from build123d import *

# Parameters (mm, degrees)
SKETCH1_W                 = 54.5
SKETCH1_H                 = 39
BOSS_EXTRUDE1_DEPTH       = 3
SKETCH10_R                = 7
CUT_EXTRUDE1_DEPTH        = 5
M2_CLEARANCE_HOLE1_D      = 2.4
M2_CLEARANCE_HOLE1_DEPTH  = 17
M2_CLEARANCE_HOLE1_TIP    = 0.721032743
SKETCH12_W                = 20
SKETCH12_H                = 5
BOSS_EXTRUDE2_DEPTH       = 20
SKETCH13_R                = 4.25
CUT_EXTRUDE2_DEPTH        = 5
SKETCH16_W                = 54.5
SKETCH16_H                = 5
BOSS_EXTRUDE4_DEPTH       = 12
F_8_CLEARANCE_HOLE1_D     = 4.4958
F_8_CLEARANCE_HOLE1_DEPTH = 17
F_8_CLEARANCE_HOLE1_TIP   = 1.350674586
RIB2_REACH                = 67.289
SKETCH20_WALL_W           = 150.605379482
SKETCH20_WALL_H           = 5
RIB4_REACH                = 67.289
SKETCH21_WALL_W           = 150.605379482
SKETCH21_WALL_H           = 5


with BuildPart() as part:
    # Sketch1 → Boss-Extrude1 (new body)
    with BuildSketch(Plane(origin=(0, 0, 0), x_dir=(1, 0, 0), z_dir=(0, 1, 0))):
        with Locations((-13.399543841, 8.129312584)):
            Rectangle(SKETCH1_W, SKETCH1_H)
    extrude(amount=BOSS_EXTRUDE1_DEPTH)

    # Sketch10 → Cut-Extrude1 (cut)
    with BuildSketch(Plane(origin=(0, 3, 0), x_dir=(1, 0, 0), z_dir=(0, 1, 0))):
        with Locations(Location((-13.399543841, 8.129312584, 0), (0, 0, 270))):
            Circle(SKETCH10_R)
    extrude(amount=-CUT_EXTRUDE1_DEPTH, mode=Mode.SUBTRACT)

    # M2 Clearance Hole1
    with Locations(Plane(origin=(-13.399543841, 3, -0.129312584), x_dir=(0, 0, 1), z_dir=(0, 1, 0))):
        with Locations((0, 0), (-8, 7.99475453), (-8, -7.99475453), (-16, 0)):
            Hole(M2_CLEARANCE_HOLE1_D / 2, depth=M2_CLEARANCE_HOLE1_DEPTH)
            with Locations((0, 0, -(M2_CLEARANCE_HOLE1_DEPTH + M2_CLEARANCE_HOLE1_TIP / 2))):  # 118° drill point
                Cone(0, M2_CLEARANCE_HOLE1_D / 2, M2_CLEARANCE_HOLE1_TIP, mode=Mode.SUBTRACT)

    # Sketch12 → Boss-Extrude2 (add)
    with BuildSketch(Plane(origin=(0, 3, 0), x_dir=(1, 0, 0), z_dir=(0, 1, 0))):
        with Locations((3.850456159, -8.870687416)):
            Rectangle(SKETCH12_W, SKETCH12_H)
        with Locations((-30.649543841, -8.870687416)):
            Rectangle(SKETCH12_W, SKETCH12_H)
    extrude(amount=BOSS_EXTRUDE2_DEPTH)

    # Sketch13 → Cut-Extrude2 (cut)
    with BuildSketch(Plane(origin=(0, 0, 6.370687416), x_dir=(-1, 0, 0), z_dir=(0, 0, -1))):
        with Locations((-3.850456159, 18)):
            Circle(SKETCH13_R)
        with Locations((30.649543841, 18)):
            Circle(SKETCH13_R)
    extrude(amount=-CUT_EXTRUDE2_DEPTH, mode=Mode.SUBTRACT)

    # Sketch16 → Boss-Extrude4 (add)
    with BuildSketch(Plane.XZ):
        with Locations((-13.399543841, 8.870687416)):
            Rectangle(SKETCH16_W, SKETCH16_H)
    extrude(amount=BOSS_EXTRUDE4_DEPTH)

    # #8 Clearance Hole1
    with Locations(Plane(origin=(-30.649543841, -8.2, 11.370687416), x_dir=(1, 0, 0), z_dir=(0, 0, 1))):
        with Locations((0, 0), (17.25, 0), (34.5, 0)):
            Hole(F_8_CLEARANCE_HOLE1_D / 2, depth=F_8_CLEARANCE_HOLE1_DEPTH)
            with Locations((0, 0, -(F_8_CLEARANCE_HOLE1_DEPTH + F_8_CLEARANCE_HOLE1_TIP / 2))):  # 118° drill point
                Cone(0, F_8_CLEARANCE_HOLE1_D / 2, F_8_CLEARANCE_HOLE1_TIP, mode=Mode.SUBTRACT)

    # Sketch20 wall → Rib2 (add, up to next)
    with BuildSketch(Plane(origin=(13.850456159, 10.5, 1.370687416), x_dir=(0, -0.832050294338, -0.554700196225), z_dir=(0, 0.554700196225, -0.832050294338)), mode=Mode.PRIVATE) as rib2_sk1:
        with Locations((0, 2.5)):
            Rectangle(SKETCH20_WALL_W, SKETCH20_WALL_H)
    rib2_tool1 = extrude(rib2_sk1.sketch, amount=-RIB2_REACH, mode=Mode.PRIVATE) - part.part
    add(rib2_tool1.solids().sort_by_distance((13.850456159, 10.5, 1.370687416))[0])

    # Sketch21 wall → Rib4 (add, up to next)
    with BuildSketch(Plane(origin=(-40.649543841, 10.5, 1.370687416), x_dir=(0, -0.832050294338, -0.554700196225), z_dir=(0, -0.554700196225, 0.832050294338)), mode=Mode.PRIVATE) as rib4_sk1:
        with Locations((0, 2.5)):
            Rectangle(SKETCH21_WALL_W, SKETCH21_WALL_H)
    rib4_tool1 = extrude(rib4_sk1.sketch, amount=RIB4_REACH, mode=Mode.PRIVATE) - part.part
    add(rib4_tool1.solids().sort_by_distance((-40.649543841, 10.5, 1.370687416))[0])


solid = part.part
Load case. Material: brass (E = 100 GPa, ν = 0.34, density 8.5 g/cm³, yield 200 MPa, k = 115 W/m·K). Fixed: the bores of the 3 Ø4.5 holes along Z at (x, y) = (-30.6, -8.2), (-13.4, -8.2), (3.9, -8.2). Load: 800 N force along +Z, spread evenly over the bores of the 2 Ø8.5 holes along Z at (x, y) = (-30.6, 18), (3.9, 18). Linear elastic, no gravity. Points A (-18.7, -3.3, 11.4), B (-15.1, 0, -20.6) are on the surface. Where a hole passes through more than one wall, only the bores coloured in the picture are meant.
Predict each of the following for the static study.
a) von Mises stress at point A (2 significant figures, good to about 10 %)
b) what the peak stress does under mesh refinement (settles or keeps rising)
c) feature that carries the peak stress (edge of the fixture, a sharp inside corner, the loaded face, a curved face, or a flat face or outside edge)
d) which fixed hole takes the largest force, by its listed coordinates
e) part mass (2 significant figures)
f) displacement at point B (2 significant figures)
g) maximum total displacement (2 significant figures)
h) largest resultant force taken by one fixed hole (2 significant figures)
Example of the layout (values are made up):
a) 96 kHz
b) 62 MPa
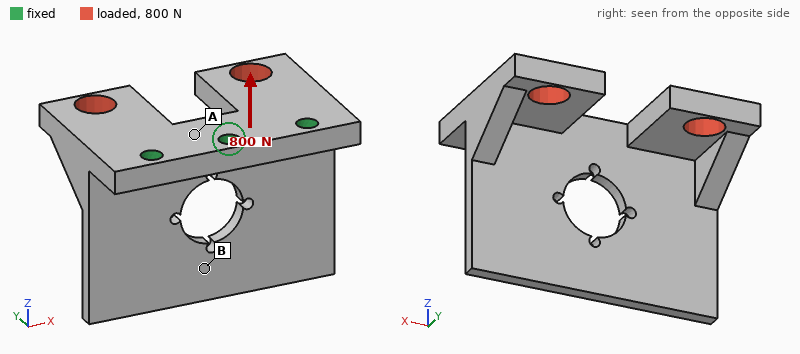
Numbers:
a) 47 MPa
b) keeps rising
c) edge of the fixture
d) (-13.4, -8.2)
e) 110 g
f) 0.094 mm
g) 0.13 mm
h) 370 N
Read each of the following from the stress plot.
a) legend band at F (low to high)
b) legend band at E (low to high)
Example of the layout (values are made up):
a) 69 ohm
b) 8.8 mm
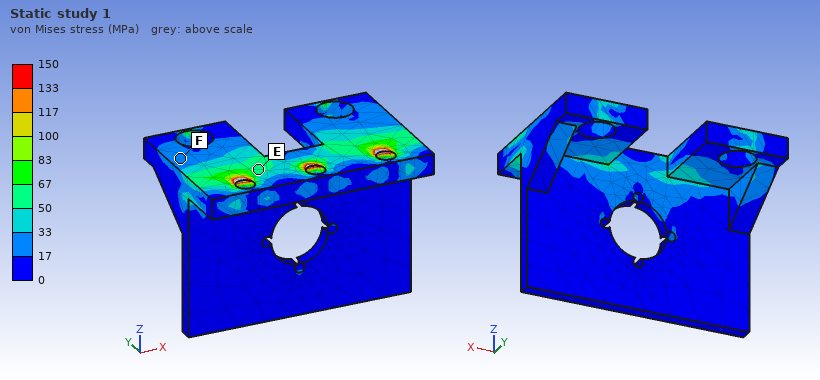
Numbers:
a) 17 to 33 MPa
b) 50 to 67 MPa
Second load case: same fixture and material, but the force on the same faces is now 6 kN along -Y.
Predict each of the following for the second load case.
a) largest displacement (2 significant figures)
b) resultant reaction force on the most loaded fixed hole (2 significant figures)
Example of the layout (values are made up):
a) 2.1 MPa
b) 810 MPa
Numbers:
a) 29 µm
b) 2.6 kN
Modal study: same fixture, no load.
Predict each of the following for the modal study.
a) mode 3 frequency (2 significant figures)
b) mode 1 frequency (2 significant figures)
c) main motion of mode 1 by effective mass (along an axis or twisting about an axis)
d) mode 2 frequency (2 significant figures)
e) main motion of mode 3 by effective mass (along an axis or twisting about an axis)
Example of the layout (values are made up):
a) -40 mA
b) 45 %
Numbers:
a) 3800 Hz
b) 1400 Hz
c) along Y
d) 2400 Hz
e) along Z
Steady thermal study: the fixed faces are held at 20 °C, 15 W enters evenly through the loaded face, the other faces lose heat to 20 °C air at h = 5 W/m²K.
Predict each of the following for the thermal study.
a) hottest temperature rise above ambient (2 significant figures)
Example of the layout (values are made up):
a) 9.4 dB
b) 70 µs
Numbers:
a) 20 K
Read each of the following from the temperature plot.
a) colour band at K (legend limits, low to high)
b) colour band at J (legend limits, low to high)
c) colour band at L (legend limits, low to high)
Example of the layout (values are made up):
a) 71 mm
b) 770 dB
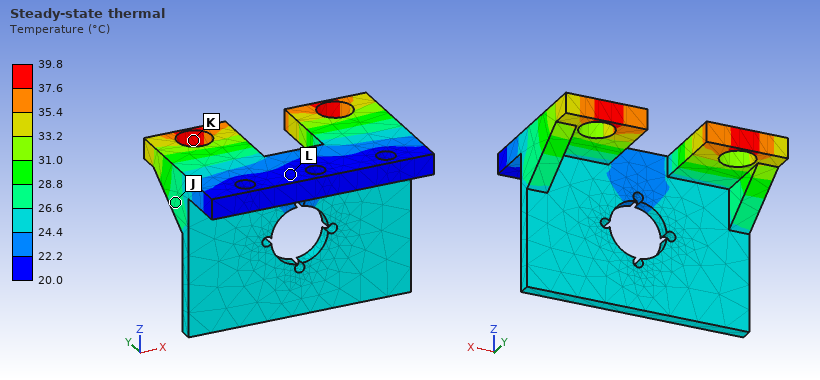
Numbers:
a) 37.6 to 39.8 °C
b) 26.6 to 28.8 °C
c) 20.0 to 22.2 °C
